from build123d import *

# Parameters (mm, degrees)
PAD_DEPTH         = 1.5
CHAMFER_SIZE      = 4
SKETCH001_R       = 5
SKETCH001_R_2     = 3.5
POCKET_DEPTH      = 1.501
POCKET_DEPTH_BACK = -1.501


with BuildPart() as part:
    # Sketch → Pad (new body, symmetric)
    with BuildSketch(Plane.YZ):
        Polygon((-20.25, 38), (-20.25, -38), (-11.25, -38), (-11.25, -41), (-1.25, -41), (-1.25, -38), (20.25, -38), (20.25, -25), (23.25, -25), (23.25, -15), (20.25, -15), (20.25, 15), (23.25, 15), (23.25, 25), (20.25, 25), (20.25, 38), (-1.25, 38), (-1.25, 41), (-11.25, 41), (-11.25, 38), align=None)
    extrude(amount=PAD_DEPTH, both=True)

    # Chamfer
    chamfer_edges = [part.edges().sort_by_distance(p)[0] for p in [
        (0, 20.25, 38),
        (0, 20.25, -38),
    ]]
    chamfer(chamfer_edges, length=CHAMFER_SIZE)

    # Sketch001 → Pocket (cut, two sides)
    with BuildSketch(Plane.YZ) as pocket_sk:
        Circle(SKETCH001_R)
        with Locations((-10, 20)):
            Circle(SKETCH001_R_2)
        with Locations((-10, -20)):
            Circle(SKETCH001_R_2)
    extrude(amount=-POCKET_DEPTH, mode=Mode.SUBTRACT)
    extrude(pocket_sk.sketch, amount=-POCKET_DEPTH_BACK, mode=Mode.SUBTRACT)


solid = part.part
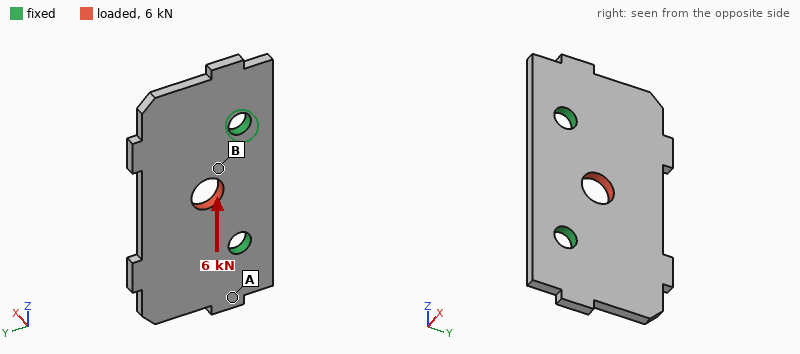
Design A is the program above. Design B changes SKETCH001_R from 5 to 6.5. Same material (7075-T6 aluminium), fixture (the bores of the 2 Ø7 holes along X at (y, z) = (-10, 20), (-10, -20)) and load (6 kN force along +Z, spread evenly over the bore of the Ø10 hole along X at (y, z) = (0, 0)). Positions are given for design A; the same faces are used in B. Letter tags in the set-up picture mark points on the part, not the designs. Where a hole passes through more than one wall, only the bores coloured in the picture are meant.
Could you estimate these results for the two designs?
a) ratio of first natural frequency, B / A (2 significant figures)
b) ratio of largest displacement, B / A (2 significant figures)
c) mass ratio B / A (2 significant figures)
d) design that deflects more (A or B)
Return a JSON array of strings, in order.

["0.99", "1.1", "0.98", "B"]
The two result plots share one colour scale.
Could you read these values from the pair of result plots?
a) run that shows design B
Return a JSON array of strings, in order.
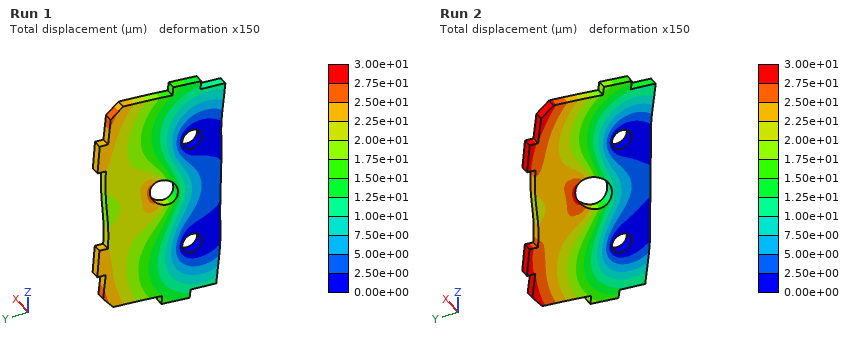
["Run 2"]
